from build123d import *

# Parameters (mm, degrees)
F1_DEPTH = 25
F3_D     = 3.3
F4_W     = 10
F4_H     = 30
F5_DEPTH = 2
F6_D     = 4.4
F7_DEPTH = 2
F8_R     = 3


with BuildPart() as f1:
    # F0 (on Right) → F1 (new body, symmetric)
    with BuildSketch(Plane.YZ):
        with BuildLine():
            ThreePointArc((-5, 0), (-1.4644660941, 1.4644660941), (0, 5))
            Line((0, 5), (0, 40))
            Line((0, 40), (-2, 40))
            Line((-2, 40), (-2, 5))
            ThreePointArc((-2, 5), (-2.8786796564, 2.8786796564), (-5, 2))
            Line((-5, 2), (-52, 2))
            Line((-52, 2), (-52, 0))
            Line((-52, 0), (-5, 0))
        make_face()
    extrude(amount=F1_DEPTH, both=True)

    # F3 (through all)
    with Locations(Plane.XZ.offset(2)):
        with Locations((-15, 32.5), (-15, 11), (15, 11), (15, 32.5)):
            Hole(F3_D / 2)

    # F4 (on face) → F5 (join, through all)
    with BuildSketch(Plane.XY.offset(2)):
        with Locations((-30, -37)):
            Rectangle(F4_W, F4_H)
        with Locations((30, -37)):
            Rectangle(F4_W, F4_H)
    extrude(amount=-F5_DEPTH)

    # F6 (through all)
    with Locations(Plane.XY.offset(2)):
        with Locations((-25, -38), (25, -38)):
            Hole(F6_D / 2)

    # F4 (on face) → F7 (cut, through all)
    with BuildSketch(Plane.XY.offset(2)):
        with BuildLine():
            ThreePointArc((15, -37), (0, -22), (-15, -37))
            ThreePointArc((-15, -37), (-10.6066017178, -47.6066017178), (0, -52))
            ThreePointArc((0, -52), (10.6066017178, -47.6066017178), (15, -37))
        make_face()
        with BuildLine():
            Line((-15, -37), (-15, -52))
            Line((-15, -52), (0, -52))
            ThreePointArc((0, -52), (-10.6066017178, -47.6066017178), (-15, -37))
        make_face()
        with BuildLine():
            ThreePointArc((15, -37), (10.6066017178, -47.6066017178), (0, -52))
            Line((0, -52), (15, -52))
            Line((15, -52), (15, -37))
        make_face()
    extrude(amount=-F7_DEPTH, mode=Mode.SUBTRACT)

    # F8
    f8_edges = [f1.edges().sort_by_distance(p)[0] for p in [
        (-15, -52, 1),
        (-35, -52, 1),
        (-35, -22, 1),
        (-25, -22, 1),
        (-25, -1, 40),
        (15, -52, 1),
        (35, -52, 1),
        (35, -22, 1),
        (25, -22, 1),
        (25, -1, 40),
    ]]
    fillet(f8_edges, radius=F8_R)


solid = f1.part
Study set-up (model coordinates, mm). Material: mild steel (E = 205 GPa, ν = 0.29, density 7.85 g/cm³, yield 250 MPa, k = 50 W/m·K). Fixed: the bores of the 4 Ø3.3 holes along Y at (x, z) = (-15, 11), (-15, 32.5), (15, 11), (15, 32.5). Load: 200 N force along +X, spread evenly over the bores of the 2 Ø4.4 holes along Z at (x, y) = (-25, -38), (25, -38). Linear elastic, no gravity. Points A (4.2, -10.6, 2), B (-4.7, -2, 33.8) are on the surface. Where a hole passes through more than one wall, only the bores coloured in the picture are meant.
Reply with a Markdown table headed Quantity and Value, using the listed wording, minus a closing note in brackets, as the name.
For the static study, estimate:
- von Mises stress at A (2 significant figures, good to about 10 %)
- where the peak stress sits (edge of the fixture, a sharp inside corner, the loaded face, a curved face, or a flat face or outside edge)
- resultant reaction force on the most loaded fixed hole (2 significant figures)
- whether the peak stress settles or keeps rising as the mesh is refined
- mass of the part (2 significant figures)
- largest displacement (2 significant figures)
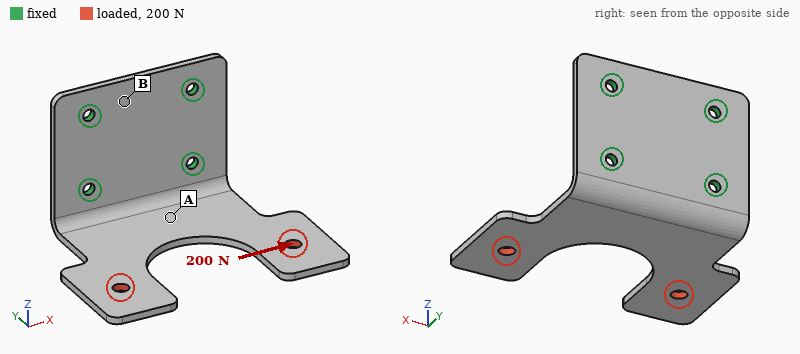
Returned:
| Quantity | Value |
|---|---|
| von Mises stress at A | 31 MPa |
| where the peak stress sits | edge of the fixture |
| resultant reaction force on the most loaded fixed hole | 270 N |
| whether the peak stress settles or keeps rising as the mesh is refined | keeps rising |
| mass of the part | 65 g |
| largest displacement | 0.11 mm |
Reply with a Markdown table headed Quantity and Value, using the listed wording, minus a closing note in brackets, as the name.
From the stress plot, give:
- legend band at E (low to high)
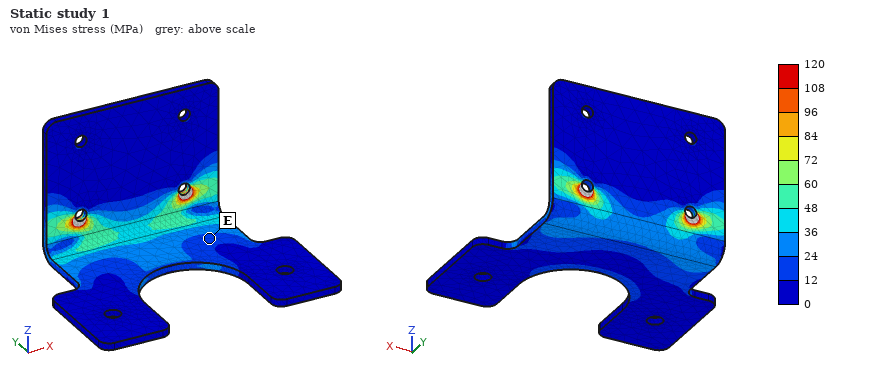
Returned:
| Quantity | Value |
|---|---|
| legend band at E | 12 to 24 MPa |
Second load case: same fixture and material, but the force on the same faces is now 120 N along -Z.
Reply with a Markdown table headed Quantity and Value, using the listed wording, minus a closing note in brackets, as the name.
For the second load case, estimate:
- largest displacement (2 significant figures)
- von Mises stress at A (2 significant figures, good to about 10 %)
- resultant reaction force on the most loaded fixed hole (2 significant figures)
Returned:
| Quantity | Value |
|---|---|
| largest displacement | 0.85 mm |
| von Mises stress at A | 79 MPa |
| resultant reaction force on the most loaded fixed hole | 54 N |
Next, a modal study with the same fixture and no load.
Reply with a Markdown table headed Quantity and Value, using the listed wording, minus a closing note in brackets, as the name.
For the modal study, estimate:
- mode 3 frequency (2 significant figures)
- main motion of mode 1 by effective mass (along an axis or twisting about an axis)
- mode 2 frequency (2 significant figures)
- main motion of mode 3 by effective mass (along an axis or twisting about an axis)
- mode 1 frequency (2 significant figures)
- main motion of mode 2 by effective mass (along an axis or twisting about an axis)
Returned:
| Quantity | Value |
|---|---|
| mode 3 frequency | 2000 Hz |
| main motion of mode 1 by effective mass | along Z |
| mode 2 frequency | 680 Hz |
| main motion of mode 3 by effective mass | along X |
| mode 1 frequency | 530 Hz |
| main motion of mode 2 by effective mass | twisting about Y |
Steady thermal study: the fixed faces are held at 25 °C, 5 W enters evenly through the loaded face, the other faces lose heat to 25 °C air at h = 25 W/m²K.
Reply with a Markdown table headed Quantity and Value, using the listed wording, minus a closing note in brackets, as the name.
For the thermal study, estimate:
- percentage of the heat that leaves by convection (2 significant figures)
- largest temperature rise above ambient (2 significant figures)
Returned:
| Quantity | Value |
|---|---|
| percentage of the heat that leaves by convection | 55 % |
| largest temperature rise above ambient | 37 K |
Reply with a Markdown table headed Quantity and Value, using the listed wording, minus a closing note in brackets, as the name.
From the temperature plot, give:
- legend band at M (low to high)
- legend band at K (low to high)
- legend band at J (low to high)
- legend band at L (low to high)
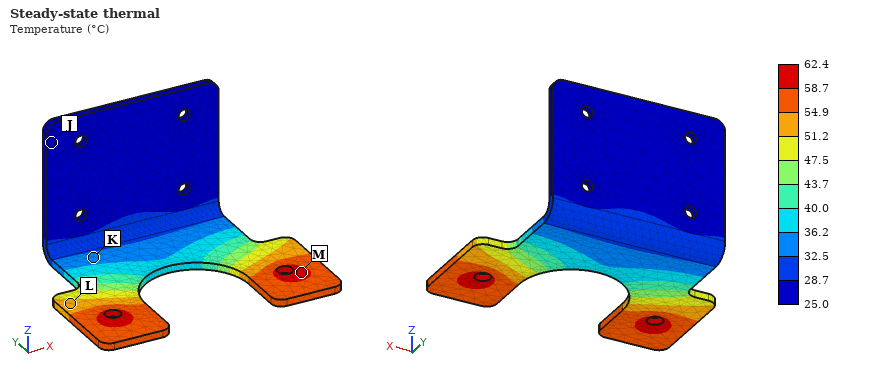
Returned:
| Quantity | Value |
|---|---|
| legend band at M | 58.7 to 62.4 °C |
| legend band at K | 32.5 to 36.2 °C |
| legend band at J | 25.0 to 28.7 °C |
| legend band at L | 51.2 to 54.9 °C |
